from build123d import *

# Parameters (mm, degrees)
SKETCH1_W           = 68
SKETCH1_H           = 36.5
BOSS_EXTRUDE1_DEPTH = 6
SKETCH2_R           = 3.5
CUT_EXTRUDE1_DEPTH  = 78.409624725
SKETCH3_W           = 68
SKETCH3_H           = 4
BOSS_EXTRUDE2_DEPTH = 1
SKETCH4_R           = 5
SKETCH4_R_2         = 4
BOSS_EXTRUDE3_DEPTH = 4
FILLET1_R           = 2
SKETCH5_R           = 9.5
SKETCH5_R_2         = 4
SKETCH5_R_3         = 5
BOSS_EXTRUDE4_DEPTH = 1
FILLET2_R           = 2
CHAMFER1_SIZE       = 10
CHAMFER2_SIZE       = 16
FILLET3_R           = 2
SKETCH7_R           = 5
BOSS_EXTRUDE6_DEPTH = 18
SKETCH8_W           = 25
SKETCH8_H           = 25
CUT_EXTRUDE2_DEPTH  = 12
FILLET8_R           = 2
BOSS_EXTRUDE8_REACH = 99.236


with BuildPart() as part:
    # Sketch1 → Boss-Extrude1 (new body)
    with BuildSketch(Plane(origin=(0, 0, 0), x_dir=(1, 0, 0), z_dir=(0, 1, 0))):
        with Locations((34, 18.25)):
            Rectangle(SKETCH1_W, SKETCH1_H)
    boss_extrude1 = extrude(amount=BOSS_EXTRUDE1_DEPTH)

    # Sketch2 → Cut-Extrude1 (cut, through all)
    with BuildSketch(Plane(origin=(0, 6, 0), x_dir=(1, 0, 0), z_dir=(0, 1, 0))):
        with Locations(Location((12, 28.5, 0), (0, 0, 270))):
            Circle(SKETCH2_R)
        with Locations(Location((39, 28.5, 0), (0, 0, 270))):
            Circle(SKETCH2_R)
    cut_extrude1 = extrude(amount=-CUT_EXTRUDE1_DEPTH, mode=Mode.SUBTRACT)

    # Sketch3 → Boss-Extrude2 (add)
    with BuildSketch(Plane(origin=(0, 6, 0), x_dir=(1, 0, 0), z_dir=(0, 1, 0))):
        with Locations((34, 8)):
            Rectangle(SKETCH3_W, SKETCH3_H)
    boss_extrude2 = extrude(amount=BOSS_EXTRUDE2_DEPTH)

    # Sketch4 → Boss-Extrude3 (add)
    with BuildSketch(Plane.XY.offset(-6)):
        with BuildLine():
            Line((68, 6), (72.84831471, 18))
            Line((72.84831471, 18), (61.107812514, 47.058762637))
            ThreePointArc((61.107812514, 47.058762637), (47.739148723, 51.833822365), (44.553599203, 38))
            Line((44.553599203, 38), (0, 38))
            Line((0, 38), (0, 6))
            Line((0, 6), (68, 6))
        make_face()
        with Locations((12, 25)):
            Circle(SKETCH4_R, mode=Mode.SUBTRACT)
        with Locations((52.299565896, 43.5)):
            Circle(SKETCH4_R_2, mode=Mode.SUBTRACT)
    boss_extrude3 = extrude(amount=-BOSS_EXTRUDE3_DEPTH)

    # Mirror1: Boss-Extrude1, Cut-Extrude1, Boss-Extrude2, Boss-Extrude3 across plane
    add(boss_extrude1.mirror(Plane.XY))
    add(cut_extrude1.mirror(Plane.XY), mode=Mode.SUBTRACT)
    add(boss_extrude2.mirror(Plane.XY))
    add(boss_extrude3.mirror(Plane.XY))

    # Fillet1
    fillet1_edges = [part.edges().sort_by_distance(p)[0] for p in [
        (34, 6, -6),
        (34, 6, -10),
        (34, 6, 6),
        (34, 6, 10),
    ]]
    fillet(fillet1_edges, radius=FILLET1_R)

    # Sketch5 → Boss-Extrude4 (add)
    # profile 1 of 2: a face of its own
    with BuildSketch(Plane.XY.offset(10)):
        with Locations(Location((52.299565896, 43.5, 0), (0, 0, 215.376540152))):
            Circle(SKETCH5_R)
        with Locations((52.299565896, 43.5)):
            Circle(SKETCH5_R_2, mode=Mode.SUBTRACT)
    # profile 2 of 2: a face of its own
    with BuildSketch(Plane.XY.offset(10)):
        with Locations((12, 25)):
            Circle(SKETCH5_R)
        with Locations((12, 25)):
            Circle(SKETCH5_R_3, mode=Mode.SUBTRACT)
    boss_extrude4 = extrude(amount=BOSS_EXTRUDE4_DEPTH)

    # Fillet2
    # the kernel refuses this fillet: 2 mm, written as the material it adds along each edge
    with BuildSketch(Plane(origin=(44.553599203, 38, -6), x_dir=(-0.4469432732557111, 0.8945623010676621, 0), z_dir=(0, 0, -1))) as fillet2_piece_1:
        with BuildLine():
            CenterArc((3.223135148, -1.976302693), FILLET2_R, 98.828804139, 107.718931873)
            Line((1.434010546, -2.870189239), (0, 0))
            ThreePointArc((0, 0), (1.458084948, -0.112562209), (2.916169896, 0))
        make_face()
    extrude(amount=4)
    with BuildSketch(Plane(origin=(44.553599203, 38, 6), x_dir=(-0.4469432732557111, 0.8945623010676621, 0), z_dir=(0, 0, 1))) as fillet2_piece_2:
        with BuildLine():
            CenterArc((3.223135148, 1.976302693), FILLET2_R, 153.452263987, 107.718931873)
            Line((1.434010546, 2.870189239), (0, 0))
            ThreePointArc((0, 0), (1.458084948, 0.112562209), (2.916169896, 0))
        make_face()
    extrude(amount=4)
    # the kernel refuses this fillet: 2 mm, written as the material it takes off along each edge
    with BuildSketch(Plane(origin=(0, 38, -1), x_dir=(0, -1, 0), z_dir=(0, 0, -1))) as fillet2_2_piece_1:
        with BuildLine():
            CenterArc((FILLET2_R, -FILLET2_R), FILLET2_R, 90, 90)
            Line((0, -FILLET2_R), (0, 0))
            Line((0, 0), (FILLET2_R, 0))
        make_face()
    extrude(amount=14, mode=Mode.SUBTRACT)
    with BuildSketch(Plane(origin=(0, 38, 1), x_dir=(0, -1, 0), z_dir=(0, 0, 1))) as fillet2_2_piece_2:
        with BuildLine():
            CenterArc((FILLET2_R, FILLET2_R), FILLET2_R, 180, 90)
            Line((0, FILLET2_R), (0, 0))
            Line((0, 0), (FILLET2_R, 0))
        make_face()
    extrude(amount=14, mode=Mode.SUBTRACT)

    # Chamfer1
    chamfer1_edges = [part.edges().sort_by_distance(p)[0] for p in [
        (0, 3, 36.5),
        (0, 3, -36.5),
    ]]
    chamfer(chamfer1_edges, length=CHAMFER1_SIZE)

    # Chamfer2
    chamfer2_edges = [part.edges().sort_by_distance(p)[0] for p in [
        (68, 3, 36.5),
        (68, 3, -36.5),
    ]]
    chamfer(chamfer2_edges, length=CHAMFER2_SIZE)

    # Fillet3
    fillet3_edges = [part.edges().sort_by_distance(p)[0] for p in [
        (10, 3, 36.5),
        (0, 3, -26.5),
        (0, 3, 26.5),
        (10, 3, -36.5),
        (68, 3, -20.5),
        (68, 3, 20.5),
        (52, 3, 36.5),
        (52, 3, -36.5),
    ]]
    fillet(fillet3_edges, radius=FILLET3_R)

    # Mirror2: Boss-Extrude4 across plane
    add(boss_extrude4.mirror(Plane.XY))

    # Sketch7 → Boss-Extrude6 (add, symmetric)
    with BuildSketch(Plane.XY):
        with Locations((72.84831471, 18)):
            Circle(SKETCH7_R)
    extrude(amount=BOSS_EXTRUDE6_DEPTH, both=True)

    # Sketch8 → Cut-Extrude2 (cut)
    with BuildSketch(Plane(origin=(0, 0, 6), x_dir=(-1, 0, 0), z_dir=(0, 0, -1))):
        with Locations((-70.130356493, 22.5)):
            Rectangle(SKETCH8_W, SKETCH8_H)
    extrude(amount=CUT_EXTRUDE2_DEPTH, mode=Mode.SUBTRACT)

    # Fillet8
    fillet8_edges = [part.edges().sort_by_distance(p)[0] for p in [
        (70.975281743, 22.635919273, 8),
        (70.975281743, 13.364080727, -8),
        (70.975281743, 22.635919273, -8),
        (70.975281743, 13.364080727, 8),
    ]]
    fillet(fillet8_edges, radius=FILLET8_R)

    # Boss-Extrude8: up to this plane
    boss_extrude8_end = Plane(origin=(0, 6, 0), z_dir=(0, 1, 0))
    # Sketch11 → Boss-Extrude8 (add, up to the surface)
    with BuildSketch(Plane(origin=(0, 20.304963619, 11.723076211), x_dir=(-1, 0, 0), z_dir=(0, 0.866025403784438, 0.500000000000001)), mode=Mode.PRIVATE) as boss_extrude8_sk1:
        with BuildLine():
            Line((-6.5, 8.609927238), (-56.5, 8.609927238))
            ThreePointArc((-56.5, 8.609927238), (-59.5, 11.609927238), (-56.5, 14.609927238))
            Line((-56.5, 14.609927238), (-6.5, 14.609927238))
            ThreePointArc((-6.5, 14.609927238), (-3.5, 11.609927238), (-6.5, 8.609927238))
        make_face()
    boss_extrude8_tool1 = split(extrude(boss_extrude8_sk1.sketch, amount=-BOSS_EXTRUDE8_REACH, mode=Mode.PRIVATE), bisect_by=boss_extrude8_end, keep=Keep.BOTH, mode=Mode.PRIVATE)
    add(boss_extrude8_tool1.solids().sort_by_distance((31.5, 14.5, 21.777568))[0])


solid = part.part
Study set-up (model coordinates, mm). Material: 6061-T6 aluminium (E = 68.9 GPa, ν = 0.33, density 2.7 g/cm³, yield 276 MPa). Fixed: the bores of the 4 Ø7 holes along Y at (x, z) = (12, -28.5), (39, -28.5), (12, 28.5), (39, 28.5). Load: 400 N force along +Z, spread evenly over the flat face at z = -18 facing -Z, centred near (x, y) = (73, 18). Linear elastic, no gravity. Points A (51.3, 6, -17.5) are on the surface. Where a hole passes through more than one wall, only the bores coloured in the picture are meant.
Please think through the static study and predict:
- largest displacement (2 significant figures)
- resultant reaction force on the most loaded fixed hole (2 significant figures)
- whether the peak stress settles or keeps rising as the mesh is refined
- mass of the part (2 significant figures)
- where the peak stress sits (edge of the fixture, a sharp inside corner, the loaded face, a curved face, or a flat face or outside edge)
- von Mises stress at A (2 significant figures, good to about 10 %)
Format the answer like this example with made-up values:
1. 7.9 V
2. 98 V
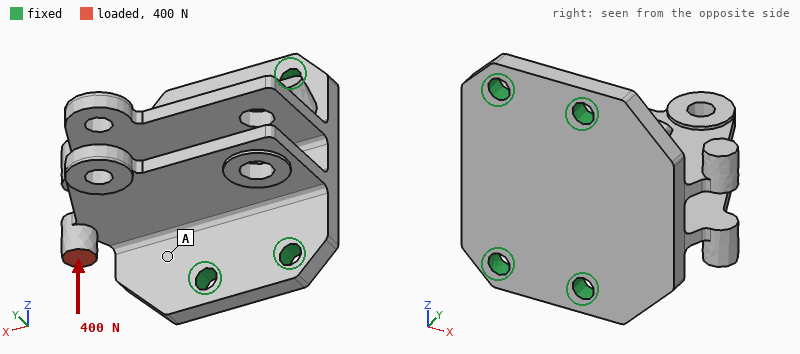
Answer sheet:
1. 0.14 mm
2. 340 N
3. keeps rising
4. 140 g
5. a sharp inside corner
6. 10 MPa
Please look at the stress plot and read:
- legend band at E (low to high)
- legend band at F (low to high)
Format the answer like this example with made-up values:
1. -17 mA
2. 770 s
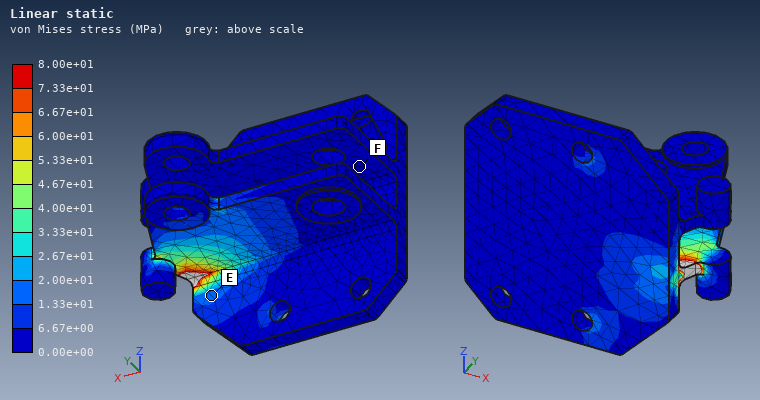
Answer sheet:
1. 1.33e+01 to 2.00e+01 MPa
2. 0.00e+00 to 6.67e+00 MPa
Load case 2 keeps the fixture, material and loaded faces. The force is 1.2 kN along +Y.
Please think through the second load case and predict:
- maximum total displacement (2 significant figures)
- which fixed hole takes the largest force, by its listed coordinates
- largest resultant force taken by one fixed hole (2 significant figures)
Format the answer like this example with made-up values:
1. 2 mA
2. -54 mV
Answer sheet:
1. 0.38 mm
2. (39, -28.5)
3. 1.6 kN
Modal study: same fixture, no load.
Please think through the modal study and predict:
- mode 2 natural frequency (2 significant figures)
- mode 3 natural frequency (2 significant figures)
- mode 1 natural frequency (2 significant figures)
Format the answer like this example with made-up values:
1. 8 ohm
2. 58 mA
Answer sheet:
1. 2200 Hz
2. 3400 Hz
3. 2100 Hz
